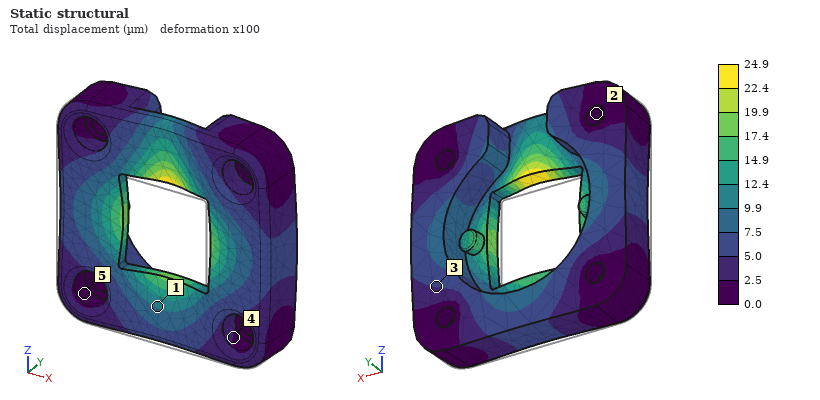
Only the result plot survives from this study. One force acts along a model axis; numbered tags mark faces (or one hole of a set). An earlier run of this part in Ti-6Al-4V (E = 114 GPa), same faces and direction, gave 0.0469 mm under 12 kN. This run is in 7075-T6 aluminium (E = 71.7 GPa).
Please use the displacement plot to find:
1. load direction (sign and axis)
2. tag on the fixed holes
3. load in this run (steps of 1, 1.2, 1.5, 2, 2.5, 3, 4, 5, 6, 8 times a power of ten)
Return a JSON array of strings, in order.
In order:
["+Y", "2", "4 kN"]
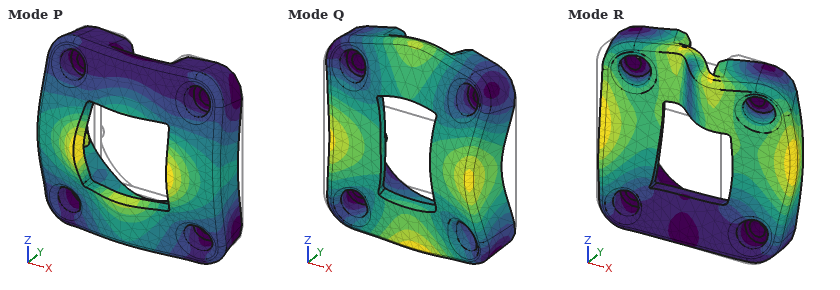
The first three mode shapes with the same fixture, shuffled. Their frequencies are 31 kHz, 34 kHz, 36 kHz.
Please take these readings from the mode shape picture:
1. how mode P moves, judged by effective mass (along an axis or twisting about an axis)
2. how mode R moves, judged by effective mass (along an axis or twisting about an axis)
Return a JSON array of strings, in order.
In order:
["along Y", "along X"]
